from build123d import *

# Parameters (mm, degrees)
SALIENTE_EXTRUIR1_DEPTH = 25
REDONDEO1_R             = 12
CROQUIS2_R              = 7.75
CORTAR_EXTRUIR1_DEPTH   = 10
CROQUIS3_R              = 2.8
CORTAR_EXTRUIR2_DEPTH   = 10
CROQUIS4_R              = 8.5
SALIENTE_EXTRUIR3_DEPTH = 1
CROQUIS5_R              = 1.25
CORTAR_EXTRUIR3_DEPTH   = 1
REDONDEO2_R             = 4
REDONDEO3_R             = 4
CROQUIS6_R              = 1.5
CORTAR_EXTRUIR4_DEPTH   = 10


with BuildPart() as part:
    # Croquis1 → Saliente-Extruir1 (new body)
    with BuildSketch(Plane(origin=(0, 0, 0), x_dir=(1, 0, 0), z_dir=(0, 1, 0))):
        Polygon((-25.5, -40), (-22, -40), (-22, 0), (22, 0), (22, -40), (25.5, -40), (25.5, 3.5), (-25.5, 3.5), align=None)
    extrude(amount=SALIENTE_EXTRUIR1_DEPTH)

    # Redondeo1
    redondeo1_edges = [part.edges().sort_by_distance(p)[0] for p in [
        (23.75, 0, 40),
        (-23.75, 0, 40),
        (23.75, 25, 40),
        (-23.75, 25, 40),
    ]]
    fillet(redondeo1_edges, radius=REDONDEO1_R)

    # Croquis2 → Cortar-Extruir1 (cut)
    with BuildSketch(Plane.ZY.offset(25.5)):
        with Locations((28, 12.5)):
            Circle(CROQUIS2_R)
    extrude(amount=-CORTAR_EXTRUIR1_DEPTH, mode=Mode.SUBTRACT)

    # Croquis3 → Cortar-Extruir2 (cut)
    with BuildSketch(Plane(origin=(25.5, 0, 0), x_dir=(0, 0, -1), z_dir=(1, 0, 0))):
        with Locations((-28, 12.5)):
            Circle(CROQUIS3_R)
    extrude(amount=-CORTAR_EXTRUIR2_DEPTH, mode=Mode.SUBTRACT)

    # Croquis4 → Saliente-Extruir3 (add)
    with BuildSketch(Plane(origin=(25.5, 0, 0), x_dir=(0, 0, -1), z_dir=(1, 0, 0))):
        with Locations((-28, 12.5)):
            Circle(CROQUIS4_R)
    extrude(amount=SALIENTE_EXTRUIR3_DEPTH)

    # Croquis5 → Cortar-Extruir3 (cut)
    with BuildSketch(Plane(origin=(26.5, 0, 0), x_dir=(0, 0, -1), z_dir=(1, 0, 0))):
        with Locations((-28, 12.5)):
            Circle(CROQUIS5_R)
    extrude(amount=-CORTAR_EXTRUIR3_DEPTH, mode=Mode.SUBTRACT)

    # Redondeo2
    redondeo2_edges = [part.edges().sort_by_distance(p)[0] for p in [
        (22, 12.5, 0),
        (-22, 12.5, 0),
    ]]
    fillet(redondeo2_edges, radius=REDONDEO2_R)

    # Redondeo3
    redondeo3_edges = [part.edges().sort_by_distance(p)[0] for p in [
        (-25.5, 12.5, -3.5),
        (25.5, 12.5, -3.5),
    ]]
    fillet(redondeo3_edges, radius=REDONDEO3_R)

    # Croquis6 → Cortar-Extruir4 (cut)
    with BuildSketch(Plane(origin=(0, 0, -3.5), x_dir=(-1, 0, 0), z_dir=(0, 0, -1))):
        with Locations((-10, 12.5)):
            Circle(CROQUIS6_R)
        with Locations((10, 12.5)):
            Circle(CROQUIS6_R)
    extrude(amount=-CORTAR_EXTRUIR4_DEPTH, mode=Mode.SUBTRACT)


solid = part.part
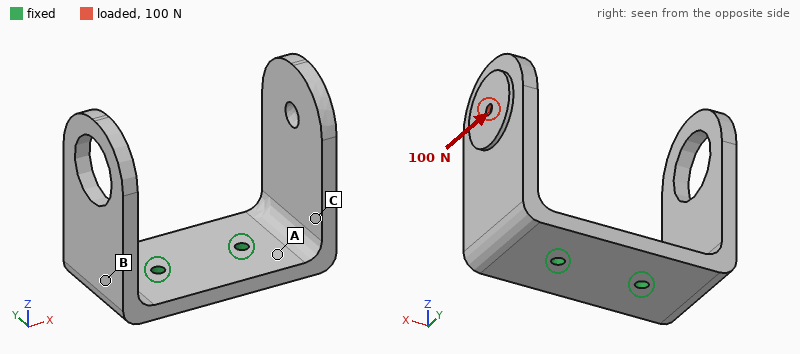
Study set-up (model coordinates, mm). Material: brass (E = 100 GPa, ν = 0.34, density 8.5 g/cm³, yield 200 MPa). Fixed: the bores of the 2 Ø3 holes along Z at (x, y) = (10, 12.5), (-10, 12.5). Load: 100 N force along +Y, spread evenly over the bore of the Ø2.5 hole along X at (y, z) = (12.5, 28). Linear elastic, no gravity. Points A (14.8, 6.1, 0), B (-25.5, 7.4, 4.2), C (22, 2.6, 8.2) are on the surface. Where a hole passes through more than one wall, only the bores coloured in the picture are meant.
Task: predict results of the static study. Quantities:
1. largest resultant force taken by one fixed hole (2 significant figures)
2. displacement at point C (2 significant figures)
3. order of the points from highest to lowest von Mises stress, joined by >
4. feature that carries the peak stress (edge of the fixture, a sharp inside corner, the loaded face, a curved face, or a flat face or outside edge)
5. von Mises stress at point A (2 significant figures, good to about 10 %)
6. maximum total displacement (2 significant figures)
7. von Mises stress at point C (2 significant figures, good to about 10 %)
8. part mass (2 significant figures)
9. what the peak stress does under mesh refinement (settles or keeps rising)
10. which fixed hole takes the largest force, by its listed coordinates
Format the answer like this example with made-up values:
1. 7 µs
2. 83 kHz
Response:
1. 170 N
2. 0.037 mm
3. A > C > B
4. edge of the fixture
5. 28 MPa
6. 0.11 mm
7. 12 MPa
8. 89 g
9. keeps rising
10. (10, 12.5)
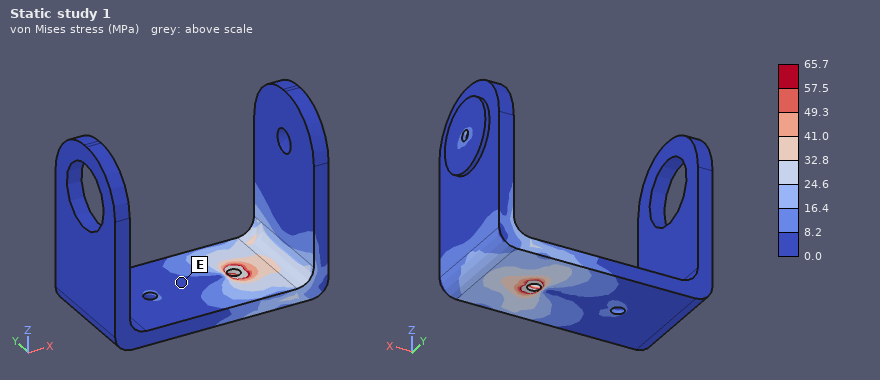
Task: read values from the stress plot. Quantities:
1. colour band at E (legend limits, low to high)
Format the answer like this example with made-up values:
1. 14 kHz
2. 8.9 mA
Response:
1. 0.0 to 8.2 MPa
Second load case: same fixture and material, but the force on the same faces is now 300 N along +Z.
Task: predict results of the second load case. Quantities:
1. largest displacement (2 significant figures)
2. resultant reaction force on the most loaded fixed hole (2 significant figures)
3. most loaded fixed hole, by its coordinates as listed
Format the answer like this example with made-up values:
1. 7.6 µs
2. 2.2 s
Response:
1. 0.23 mm
2. 390 N
3. (10, 12.5)
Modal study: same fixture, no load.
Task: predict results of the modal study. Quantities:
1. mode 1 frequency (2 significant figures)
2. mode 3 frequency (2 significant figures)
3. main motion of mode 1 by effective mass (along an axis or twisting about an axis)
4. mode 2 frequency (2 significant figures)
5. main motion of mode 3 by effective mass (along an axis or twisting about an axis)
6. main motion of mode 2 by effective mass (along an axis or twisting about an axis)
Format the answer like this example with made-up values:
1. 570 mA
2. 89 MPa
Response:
1. 840 Hz
2. 1300 Hz
3. along X
4. 1000 Hz
5. along Y
6. along X
